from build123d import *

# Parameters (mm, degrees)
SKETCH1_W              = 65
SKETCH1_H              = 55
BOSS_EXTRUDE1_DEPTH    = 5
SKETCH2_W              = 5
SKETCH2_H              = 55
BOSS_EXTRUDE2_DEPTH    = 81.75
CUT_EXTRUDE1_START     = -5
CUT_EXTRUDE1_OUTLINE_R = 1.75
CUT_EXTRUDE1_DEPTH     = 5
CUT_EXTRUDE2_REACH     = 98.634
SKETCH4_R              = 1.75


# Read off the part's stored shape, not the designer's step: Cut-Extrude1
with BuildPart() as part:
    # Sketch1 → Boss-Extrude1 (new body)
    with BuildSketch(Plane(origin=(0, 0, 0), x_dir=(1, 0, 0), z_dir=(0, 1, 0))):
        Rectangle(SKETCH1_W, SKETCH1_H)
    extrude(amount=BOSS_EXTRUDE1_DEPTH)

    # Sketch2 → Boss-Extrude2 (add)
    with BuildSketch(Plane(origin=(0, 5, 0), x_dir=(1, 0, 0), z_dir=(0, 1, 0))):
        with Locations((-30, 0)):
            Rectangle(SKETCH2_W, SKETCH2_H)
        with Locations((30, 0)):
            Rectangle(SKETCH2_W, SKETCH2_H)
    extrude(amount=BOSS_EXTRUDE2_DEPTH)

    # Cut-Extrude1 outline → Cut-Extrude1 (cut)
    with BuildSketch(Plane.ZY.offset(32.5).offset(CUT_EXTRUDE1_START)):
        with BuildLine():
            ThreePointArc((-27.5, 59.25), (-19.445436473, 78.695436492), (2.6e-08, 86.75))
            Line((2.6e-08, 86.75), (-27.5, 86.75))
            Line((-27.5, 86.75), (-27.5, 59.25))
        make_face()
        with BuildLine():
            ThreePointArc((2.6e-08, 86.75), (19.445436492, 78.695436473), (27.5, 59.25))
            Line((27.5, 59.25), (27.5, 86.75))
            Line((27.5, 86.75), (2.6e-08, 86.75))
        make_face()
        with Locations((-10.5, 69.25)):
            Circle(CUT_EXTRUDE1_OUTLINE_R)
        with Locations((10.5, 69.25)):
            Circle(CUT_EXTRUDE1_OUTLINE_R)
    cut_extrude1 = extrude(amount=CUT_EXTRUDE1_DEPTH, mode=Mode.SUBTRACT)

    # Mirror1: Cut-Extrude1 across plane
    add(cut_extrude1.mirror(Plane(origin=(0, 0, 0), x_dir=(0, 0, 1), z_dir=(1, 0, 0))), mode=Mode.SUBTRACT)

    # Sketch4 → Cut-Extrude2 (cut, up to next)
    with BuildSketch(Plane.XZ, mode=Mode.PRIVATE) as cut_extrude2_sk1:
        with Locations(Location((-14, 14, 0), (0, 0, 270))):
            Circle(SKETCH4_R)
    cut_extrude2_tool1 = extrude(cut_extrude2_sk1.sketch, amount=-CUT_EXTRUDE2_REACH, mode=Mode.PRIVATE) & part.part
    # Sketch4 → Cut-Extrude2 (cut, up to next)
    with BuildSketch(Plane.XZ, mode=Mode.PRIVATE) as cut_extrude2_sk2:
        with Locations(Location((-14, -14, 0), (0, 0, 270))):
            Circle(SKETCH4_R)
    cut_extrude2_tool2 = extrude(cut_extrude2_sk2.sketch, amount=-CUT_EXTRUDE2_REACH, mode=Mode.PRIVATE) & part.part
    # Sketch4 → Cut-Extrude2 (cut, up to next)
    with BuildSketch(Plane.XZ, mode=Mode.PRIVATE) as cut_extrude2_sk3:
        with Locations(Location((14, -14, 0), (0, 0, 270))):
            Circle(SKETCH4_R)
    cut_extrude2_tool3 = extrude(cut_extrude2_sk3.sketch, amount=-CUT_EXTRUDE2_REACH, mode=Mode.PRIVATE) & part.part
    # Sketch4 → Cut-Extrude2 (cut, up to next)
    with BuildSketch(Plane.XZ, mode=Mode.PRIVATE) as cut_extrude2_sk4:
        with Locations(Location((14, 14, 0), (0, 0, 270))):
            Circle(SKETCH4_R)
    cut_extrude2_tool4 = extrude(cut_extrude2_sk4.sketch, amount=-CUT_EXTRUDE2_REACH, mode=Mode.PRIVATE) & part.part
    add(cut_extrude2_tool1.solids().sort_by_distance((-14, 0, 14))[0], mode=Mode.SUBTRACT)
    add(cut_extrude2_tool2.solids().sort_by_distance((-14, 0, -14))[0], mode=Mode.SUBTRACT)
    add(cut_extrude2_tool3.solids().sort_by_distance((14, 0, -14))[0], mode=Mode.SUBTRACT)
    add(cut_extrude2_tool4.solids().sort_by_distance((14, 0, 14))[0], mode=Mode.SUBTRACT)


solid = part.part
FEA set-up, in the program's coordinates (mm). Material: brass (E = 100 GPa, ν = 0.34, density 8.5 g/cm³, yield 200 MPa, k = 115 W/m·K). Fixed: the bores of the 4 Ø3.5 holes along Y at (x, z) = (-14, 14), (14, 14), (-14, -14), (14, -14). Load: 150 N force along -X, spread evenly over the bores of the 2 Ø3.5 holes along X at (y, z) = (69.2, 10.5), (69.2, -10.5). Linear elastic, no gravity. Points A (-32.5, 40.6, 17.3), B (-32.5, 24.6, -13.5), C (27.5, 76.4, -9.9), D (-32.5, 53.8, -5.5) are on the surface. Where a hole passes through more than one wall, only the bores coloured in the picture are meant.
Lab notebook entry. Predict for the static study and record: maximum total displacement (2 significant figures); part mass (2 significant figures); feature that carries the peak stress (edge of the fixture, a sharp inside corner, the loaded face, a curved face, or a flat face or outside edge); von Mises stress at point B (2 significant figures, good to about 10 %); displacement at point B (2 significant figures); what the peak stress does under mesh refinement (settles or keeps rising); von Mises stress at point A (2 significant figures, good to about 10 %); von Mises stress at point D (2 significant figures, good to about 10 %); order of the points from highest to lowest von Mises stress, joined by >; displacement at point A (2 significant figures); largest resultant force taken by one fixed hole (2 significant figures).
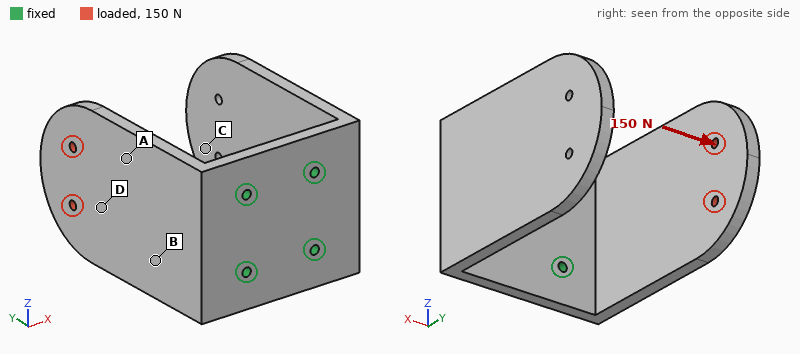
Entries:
0.56 mm
500 g
edge of the fixture
27 MPa
0.10 mm
keeps rising
18 MPa
11 MPa
B > A > D > C
0.20 mm
100 N
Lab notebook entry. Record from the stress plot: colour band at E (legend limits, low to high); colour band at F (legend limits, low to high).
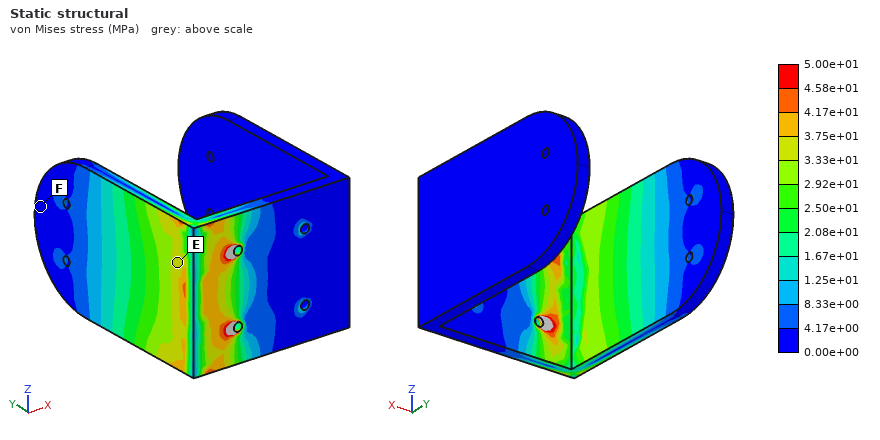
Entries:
3.33e+01 to 3.75e+01 MPa
0.00e+00 to 4.17e+00 MPa
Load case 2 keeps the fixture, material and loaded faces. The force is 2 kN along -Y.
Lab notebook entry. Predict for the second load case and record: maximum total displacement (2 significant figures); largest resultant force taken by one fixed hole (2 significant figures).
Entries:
0.43 mm
1.2 kN
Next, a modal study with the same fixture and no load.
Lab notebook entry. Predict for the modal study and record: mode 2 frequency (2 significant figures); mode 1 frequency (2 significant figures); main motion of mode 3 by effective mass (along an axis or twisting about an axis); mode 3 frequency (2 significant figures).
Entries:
340 Hz
340 Hz
along Z
950 Hz
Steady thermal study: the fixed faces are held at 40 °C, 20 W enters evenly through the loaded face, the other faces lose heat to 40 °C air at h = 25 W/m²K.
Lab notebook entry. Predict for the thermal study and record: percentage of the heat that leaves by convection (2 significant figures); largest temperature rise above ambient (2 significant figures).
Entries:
33 %
44 K
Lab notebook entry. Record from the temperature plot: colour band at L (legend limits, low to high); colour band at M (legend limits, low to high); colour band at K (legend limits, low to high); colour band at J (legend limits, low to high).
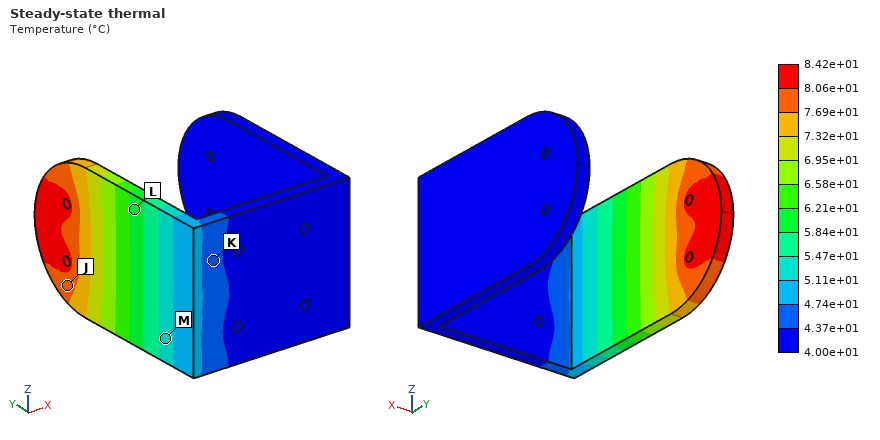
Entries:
5.84e+01 to 6.21e+01 °C
5.11e+01 to 5.47e+01 °C
4.37e+01 to 4.74e+01 °C
7.69e+01 to 8.06e+01 °C
